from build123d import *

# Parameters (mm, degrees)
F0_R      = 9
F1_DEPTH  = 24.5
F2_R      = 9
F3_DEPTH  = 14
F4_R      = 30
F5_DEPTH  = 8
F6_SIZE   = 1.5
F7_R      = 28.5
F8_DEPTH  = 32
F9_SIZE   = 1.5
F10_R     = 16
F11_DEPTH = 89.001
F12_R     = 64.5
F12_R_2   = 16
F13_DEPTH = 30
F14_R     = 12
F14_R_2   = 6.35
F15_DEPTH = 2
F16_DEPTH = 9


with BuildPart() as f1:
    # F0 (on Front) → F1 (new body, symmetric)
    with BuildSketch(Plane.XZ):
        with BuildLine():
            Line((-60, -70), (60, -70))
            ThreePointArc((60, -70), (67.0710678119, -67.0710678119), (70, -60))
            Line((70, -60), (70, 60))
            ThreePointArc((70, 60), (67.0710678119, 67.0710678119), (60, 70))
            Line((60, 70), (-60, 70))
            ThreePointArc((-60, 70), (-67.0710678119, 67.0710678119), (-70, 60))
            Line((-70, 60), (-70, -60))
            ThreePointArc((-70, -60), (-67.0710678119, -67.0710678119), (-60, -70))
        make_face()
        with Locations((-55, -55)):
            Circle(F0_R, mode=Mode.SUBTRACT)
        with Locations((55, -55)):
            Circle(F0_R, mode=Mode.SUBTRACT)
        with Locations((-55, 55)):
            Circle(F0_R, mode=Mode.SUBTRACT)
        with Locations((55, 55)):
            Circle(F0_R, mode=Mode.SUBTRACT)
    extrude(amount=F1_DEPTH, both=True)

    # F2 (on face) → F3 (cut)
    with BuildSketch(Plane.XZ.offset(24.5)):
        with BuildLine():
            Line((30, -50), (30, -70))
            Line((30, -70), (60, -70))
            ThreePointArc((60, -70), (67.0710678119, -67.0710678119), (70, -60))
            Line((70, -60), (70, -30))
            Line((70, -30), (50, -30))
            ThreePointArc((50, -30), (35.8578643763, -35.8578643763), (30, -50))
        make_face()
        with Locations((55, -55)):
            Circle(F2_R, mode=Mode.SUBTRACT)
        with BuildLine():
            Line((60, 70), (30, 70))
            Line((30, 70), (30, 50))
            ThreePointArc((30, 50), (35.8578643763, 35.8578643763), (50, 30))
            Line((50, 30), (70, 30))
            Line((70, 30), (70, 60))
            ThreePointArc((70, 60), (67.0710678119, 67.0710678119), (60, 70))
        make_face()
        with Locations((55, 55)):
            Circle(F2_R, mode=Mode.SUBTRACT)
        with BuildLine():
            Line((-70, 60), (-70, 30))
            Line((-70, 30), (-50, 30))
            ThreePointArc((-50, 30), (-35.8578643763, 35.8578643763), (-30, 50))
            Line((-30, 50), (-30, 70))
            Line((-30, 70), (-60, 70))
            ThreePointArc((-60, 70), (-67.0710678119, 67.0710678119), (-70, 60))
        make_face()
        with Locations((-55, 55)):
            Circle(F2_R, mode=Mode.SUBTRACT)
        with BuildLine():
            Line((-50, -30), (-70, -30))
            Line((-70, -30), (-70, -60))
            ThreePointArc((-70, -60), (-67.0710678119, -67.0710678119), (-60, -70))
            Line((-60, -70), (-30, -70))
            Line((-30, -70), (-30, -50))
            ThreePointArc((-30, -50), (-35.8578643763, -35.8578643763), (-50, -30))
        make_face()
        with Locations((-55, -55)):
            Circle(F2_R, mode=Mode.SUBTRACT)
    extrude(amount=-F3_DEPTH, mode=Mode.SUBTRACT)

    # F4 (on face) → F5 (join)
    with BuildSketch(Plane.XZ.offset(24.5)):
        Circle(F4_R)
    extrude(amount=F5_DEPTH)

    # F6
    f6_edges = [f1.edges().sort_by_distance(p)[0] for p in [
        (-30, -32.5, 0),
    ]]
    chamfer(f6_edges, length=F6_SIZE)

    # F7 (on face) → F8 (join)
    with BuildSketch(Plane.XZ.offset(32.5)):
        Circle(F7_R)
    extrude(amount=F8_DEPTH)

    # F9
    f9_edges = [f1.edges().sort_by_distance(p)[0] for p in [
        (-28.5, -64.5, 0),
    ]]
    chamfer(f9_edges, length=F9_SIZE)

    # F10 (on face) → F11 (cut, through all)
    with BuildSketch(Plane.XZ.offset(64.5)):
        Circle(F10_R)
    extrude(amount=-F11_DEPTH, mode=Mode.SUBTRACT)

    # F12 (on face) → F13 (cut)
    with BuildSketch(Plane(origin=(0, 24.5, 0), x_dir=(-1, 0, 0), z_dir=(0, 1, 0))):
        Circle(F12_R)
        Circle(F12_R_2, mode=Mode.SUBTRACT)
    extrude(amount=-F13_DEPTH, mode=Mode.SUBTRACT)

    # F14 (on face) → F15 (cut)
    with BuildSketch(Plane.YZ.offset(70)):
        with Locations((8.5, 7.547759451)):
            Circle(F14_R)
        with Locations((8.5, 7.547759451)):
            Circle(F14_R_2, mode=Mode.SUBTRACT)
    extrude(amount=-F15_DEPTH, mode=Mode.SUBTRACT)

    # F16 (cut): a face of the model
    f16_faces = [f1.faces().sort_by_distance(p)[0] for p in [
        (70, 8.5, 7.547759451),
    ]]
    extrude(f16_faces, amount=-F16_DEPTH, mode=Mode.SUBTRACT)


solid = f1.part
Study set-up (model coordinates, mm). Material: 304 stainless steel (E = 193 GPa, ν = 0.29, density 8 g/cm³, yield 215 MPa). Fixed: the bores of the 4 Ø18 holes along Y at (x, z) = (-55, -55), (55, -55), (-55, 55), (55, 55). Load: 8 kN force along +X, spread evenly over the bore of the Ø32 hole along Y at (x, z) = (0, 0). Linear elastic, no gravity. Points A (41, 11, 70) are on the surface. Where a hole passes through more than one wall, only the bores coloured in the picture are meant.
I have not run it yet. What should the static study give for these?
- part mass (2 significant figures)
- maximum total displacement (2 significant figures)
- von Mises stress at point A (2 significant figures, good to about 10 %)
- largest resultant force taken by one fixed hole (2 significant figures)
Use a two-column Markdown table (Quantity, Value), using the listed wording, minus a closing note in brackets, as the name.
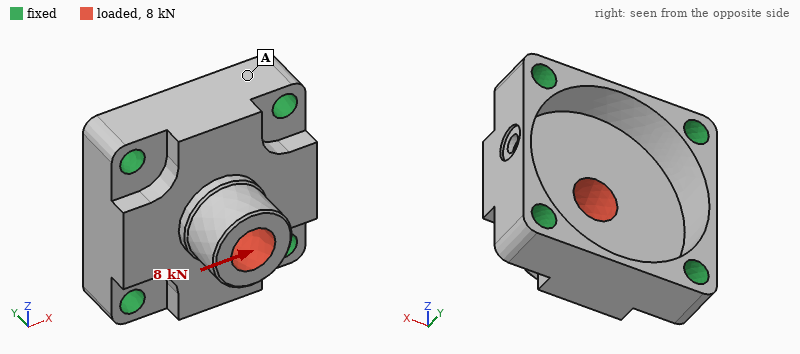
| Quantity | Value |
|---|---|
| part mass | 4.0 kg |
| maximum total displacement | 6.6 µm |
| von Mises stress at point A | 1.9 MPa |
| largest resultant force taken by one fixed hole | 2.5 kN |
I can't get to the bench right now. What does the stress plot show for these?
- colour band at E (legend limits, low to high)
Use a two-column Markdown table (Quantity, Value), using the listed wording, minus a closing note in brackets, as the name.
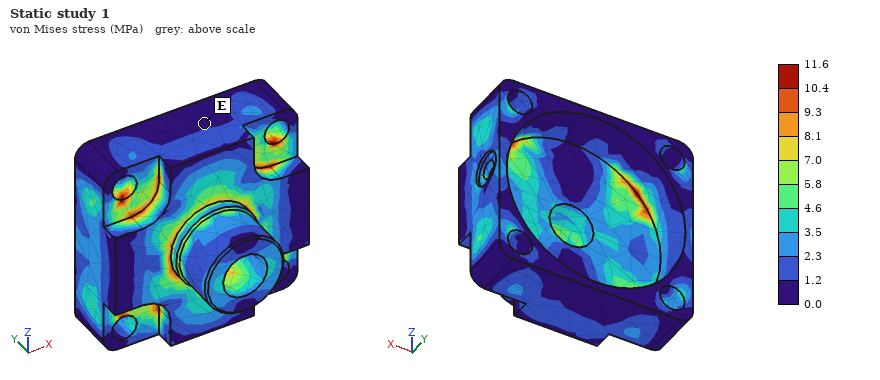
| Quantity | Value |
|---|---|
| colour band at E | 0.0 to 1.2 MPa |
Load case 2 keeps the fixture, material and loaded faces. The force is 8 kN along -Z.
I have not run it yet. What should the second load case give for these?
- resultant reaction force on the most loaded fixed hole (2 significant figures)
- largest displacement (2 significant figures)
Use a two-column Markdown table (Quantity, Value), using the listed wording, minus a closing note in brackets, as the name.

| Quantity | Value |
|---|---|
| resultant reaction force on the most loaded fixed hole | 2.5 kN |
| largest displacement | 6.5 µm |
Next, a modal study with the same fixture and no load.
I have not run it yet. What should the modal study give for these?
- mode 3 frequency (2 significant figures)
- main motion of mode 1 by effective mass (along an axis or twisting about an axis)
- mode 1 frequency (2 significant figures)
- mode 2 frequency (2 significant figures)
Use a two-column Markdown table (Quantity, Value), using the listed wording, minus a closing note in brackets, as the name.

| Quantity | Value |
|---|---|
| mode 3 frequency | 6200 Hz |
| main motion of mode 1 by effective mass | along Y |
| mode 1 frequency | 4700 Hz |
| mode 2 frequency | 6200 Hz |
